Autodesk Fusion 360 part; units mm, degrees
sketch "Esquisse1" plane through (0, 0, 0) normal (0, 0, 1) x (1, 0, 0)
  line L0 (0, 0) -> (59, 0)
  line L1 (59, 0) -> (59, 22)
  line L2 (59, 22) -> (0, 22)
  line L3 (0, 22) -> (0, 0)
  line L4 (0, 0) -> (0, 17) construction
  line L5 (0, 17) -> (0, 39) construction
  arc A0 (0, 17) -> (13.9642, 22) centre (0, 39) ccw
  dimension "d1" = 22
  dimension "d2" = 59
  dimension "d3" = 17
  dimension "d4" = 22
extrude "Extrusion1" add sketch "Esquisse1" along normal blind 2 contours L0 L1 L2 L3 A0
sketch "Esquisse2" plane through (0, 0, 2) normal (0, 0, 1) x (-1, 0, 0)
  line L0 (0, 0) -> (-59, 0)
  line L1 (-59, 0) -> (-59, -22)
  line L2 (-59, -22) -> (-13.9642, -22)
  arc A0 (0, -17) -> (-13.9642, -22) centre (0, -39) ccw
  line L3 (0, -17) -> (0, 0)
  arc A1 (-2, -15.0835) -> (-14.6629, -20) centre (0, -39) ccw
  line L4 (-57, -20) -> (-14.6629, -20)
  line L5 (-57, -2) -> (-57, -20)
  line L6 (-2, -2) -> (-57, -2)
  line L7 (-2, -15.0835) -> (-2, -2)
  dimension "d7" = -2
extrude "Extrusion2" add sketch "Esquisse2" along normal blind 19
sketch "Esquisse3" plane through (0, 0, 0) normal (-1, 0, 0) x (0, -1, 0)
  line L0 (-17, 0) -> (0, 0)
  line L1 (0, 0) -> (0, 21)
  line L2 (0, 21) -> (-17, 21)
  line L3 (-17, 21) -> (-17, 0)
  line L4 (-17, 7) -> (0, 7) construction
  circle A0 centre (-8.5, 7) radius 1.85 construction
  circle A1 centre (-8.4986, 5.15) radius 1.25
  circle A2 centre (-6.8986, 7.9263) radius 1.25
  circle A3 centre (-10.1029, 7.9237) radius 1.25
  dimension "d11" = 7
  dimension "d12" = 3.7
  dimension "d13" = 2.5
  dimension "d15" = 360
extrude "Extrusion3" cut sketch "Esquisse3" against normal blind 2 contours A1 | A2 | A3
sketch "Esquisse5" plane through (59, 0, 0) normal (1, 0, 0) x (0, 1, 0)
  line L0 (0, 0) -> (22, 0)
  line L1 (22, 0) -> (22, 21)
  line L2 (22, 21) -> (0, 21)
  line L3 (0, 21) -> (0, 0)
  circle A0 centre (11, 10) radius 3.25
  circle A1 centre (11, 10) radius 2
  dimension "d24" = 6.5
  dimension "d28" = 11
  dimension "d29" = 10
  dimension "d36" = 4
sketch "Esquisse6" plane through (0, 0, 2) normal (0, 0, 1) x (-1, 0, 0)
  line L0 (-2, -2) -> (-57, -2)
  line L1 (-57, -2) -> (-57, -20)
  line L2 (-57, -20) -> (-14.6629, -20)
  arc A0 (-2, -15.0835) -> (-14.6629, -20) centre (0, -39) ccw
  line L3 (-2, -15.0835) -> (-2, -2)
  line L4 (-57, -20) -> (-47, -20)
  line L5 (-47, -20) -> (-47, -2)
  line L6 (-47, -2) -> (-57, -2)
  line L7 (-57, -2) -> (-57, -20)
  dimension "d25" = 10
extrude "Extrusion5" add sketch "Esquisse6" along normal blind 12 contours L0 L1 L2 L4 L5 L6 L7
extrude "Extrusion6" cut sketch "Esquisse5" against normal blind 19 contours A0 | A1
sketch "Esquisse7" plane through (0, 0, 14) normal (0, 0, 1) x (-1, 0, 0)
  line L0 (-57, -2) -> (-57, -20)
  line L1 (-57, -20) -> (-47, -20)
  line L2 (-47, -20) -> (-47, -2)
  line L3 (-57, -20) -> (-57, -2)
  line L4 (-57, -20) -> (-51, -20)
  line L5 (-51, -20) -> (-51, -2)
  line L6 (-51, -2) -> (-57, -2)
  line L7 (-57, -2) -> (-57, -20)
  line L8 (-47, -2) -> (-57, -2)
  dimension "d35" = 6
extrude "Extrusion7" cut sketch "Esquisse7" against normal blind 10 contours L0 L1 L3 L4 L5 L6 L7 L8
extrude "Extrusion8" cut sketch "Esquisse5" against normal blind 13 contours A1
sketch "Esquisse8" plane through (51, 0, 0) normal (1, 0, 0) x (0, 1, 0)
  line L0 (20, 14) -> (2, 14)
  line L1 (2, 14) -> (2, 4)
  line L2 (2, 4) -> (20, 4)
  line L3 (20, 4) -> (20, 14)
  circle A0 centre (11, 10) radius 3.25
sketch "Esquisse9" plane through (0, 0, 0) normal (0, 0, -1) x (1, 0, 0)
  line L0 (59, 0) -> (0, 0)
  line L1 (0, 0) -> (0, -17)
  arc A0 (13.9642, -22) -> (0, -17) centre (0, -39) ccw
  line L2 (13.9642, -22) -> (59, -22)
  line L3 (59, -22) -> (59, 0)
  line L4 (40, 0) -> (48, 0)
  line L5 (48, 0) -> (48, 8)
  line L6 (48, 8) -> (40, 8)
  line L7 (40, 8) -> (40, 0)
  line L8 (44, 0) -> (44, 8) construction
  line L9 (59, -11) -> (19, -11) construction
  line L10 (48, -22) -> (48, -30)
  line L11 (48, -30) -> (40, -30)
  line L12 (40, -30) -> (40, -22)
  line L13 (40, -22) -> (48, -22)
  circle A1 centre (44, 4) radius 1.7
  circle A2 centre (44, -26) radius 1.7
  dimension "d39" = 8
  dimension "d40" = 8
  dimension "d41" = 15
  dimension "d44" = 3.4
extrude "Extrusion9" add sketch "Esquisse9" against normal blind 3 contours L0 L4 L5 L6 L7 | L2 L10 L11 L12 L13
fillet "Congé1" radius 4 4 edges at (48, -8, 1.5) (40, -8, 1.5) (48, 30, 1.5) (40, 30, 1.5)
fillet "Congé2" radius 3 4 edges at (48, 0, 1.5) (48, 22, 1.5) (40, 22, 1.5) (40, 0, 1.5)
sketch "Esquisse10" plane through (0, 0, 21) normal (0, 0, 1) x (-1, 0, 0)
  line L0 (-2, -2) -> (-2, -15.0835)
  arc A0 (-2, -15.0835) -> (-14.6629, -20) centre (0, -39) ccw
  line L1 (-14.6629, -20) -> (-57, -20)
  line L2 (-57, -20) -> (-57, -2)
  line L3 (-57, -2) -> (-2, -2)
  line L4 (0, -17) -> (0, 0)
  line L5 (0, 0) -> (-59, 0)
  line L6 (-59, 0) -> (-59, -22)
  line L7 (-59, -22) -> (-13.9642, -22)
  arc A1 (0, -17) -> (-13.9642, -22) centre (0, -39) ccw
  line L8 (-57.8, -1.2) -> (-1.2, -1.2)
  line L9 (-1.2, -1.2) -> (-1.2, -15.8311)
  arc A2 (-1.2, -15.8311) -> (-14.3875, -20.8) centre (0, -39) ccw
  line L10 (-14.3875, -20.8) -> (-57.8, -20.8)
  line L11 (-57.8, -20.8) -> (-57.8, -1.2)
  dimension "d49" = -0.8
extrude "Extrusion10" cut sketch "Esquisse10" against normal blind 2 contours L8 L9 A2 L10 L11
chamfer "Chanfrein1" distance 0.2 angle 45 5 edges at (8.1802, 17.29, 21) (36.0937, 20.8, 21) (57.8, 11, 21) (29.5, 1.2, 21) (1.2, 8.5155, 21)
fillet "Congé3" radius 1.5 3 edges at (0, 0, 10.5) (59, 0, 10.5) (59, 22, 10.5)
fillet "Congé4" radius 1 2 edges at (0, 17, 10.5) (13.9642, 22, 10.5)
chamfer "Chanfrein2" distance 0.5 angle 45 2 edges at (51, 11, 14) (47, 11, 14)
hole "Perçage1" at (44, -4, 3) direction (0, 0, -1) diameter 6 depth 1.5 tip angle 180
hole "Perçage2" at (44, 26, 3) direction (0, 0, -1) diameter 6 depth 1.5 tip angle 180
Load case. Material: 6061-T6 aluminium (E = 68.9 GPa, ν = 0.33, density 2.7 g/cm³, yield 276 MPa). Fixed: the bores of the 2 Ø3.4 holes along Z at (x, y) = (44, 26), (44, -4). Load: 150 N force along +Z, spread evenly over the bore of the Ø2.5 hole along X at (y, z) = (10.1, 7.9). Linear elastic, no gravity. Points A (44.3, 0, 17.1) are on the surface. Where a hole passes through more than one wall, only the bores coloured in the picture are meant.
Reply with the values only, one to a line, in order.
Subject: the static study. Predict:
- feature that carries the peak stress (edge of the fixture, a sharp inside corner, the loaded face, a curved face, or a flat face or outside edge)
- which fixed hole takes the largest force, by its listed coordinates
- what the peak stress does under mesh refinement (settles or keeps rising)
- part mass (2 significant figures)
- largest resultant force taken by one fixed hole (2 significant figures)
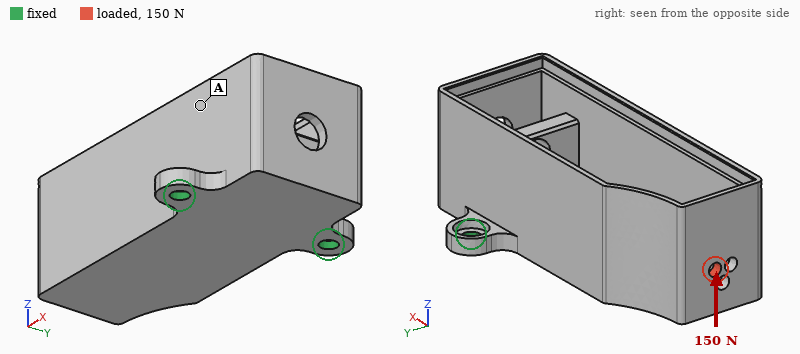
edge of the fixture
(44, -4)
keeps rising
24 g
81 N
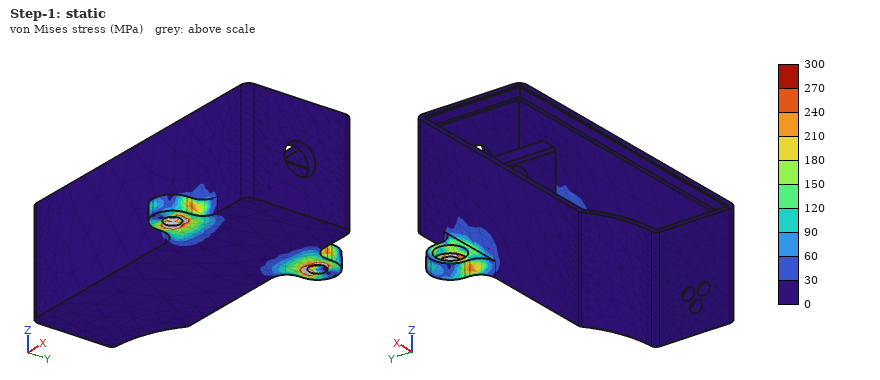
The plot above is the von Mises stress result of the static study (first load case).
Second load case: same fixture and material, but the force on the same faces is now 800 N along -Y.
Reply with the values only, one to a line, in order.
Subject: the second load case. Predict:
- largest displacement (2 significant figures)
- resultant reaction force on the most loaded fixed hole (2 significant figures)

0.46 mm
1.3 kN
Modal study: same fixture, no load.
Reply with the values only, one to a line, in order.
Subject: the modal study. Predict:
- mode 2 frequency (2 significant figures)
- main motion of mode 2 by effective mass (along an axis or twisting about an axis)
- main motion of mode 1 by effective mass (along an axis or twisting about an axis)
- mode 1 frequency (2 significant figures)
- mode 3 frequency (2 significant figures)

2800 Hz
along Y
along Z
950 Hz
5700 Hz
